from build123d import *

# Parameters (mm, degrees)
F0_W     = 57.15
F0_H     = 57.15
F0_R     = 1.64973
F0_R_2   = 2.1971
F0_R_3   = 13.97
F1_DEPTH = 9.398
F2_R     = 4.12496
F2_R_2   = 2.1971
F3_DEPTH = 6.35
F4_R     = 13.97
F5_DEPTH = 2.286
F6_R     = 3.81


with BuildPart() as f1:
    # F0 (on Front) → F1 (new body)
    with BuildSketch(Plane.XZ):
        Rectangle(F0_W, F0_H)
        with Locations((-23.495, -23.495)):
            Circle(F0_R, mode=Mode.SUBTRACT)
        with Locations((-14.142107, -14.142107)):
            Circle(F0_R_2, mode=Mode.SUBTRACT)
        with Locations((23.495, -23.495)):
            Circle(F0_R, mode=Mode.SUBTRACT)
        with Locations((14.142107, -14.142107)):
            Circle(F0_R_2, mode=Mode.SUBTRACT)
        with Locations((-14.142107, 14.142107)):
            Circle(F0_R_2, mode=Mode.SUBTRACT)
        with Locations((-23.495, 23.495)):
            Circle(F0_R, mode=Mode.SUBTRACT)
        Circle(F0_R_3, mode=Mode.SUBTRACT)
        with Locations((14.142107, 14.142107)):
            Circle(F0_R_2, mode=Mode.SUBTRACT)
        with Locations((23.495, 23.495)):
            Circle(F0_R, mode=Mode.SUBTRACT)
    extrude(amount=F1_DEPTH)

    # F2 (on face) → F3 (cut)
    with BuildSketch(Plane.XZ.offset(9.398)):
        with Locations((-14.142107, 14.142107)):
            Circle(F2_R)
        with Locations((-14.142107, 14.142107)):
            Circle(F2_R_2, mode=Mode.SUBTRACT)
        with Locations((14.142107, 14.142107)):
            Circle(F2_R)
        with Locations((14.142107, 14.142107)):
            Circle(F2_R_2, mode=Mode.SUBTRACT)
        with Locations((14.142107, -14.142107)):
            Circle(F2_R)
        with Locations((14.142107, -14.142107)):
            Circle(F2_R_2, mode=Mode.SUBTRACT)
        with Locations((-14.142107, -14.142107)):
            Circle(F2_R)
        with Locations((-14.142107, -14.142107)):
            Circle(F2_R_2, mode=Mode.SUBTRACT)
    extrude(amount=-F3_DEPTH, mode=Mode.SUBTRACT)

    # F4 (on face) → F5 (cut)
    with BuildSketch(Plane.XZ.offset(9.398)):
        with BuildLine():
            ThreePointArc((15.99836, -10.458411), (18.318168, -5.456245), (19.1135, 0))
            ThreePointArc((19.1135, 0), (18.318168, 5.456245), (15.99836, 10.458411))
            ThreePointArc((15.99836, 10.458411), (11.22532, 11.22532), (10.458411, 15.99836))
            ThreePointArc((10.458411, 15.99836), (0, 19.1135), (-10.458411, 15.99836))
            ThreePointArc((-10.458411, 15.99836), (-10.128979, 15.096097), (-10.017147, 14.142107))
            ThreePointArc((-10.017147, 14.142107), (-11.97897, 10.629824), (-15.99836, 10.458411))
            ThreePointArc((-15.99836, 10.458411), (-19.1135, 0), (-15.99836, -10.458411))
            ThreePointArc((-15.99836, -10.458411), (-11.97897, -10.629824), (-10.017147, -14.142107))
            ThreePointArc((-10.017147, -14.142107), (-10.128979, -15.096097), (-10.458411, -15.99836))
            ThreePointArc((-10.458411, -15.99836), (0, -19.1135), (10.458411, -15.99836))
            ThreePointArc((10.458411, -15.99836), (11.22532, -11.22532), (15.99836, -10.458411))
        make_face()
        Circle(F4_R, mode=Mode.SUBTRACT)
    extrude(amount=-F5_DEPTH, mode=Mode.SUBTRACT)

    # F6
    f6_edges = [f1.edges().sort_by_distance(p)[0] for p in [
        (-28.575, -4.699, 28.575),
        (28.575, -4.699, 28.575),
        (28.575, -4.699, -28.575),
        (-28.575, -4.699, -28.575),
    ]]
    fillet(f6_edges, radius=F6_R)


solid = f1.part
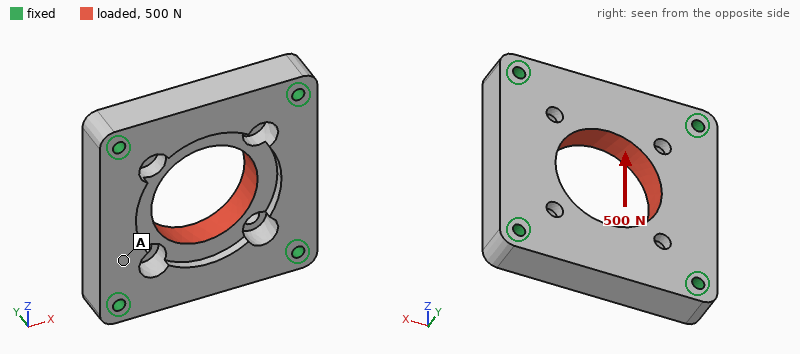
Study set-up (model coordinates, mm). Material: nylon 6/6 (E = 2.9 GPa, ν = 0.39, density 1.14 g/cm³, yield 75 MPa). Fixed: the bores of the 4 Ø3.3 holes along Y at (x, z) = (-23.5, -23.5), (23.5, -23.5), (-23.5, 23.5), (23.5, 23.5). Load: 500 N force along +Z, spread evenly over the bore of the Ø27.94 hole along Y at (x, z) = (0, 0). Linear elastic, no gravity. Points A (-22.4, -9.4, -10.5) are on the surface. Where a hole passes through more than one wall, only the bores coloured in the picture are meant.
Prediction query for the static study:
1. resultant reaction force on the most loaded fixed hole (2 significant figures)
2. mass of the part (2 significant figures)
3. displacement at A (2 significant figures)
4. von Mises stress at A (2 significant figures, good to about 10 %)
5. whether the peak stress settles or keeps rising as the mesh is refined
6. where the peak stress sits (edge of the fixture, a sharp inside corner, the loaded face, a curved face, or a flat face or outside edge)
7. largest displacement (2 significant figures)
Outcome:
140 N
25 g
4.2 µm
0.54 MPa
keeps rising
edge of the fixture
19 µm
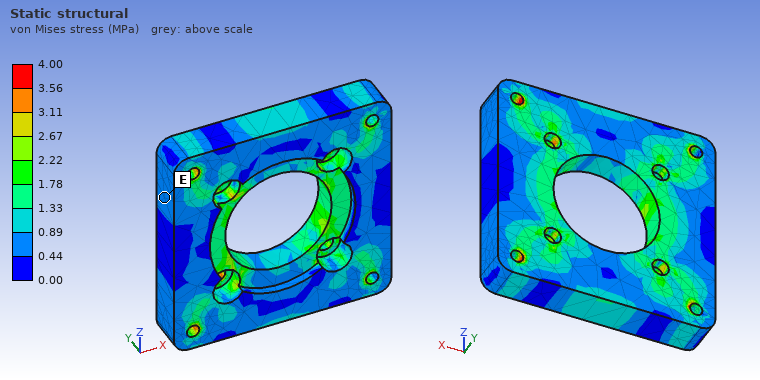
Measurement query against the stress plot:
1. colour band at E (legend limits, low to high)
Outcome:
0.44 to 0.89 MPa
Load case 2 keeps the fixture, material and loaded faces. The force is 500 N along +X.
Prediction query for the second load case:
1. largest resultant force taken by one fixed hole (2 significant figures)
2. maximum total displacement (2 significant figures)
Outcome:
140 N
19 µm
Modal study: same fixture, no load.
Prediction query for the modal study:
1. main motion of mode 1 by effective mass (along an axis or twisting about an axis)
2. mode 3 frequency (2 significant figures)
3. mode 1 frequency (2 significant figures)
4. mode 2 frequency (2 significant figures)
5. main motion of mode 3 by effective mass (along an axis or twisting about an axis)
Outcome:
along Y
5500 Hz
4400 Hz
5300 Hz
twisting about X
